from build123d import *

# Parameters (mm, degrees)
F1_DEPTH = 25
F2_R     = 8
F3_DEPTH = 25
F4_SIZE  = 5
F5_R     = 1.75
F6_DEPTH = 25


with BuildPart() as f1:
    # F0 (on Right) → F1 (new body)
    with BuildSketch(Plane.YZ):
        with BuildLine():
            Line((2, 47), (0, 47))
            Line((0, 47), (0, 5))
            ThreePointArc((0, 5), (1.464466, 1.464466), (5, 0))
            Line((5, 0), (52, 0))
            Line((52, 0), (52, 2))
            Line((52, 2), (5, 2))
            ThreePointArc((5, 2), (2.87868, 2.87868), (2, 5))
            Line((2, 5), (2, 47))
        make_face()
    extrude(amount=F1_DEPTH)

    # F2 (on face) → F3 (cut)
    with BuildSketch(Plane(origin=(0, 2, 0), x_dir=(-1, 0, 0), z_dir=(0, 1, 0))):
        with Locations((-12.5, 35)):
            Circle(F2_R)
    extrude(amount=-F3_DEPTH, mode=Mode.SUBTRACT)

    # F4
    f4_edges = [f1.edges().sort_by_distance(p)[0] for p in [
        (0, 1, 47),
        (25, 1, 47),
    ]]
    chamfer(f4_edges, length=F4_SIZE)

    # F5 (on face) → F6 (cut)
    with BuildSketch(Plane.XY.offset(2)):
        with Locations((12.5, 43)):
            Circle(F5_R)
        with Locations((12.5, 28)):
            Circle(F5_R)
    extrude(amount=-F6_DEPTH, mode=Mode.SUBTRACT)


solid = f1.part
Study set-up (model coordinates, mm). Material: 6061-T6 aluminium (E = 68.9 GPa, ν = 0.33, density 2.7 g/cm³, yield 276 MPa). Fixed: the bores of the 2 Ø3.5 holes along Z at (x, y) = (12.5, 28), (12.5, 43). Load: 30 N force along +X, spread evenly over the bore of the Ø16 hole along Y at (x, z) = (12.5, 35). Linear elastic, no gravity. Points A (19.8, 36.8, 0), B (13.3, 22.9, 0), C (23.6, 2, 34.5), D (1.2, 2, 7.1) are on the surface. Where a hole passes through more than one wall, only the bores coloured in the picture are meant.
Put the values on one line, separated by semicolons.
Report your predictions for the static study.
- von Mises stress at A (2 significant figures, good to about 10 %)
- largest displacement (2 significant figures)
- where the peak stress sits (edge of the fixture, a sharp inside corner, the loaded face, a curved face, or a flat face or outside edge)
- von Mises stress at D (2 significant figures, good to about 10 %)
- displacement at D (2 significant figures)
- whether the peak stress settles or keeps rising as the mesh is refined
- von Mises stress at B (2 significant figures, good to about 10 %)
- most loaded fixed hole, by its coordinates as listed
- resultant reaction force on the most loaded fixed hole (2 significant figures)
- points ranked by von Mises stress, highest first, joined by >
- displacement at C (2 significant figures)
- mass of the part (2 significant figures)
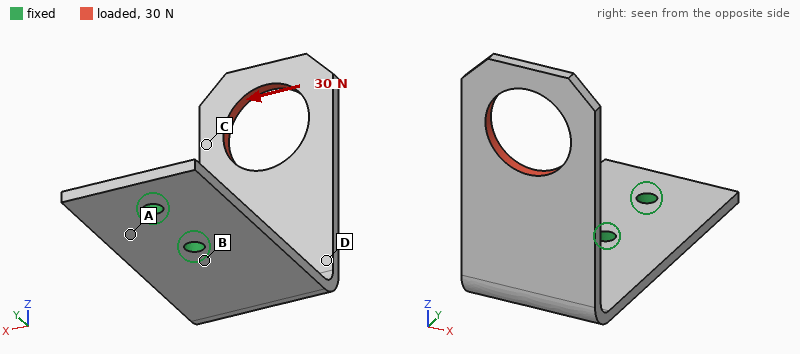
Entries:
14 MPa; 0.68 mm; edge of the fixture; 25 MPa; 0.19 mm; keeps rising; 55 MPa; (12.5, 28); 72 N; B > D > A > C; 0.52 mm; 12 g
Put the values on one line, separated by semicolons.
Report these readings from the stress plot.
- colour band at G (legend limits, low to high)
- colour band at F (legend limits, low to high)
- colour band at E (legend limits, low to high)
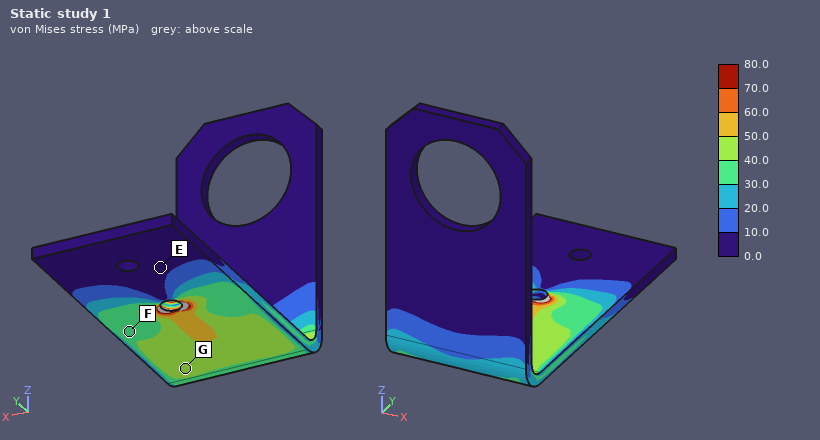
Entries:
40.0 to 50.0 MPa; 30.0 to 40.0 MPa; 0.0 to 10.0 MPa
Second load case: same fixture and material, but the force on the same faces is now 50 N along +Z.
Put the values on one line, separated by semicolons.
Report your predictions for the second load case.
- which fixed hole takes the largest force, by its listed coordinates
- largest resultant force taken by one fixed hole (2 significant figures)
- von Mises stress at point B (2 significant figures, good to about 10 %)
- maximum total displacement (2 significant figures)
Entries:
(12.5, 28); 78 N; 73 MPa; 0.77 mm
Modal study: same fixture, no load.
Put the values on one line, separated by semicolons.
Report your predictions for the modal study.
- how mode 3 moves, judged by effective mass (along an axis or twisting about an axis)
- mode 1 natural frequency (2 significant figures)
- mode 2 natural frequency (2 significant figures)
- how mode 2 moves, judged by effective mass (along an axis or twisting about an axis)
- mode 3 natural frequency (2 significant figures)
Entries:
along Z; 490 Hz; 740 Hz; along X; 1400 Hz
